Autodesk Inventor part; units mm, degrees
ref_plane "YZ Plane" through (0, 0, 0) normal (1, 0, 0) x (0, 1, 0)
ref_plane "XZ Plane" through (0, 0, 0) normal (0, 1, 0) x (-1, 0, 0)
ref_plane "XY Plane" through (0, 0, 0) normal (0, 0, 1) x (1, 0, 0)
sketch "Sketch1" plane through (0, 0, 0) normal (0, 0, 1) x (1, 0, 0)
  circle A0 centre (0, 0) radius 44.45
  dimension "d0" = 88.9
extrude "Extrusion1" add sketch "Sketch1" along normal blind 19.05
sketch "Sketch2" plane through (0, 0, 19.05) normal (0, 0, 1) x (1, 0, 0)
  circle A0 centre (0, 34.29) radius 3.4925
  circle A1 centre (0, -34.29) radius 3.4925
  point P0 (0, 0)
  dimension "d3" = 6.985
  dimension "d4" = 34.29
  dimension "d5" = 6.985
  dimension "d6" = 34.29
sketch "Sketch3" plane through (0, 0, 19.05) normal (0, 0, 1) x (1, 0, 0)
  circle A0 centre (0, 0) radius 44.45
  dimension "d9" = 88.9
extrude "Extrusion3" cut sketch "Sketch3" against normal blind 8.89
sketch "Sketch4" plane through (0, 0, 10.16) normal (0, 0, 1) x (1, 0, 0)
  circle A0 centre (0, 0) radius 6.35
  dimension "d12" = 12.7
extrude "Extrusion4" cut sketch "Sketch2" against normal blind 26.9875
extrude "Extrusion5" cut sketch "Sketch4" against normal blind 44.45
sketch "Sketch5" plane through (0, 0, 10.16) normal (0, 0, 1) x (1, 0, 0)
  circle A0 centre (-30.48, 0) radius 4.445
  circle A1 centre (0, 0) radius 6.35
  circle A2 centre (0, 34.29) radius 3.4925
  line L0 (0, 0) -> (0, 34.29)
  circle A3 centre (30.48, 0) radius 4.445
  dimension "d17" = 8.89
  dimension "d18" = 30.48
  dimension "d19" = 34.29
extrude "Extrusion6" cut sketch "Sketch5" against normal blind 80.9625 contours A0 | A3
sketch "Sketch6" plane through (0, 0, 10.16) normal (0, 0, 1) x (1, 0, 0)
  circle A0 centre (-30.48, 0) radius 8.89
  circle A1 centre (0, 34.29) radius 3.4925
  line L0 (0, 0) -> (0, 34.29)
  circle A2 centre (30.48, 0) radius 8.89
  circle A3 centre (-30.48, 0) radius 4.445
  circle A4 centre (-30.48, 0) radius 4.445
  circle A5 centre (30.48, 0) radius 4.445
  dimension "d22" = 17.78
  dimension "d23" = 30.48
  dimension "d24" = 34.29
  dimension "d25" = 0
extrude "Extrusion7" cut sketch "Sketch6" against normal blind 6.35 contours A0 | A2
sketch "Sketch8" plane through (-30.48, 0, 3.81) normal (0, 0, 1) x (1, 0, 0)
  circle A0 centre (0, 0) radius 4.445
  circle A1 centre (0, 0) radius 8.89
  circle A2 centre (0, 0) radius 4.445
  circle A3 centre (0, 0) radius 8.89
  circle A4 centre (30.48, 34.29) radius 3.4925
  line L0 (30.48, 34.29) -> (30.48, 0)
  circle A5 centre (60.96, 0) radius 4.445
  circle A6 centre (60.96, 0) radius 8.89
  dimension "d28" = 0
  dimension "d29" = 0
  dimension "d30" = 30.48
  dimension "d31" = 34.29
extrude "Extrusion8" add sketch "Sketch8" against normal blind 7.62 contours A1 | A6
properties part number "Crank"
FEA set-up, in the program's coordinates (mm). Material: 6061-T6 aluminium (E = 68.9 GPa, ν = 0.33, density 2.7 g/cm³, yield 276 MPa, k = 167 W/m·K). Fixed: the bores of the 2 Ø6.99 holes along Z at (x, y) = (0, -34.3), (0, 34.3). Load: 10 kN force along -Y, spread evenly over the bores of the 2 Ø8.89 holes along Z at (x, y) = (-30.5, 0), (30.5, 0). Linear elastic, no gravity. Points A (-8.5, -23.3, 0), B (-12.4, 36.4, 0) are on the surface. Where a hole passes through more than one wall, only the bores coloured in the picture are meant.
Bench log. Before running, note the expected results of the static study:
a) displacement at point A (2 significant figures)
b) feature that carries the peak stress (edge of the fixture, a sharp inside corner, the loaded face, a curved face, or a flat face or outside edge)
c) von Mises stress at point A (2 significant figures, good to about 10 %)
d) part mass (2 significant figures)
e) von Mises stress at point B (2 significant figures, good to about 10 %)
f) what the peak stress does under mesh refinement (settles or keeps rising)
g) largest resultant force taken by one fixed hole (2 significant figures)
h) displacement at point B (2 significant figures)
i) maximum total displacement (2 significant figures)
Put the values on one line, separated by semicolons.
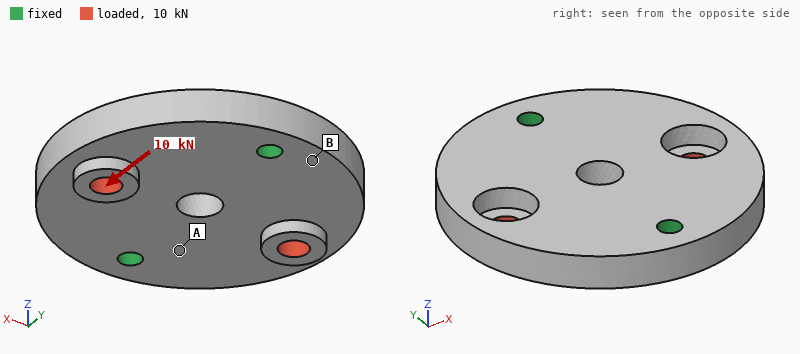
4.5 µm; edge of the fixture; 19 MPa; 160 g; 8.3 MPa; keeps rising; 5.1 kN; 4.5 µm; 24 µm
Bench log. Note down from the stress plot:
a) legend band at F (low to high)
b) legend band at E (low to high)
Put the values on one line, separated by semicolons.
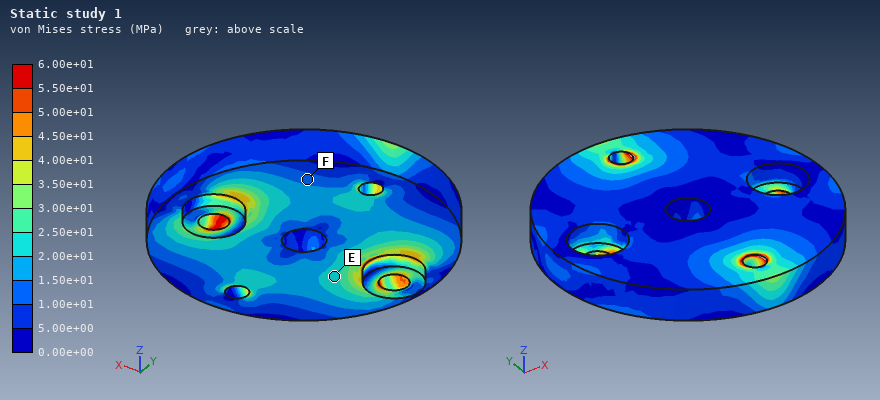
1.00e+01 to 1.50e+01 MPa; 2.00e+01 to 2.50e+01 MPa
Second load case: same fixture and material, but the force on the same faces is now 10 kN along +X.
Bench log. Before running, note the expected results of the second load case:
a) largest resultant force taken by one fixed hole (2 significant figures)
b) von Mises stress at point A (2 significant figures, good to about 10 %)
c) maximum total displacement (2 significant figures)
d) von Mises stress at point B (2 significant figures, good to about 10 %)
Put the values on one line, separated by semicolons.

5.0 kN; 34 MPa; 96 µm; 33 MPa
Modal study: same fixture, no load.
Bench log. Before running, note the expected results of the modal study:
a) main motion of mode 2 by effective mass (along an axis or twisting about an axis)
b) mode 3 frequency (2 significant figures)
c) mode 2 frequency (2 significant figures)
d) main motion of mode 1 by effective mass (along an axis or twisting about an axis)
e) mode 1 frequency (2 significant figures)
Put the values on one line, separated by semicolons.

along Z; 9300 Hz; 4700 Hz; twisting about Y; 3700 Hz
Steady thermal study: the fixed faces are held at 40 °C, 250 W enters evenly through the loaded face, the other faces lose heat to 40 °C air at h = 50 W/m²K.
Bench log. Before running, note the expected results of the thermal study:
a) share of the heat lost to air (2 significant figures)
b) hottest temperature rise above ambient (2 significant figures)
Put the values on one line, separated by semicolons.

11 %; 77 K
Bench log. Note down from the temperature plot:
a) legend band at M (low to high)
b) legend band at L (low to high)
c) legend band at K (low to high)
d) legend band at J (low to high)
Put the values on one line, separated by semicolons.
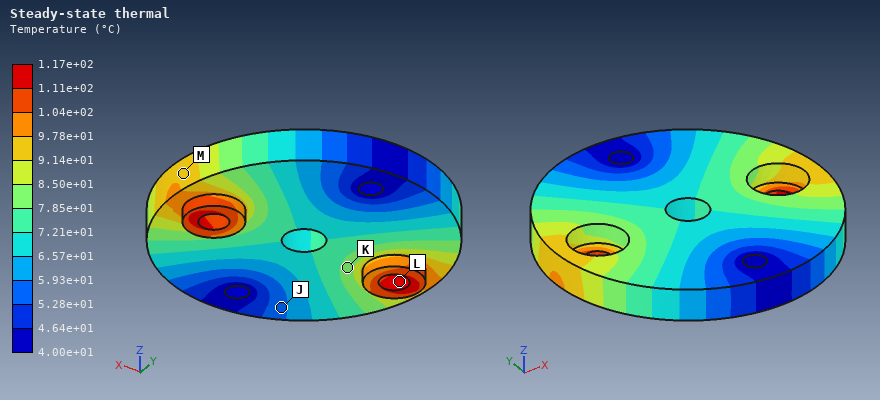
9.14e+01 to 9.78e+01 °C; 1.11e+02 to 1.17e+02 °C; 7.85e+01 to 8.50e+01 °C; 5.28e+01 to 5.93e+01 °C
